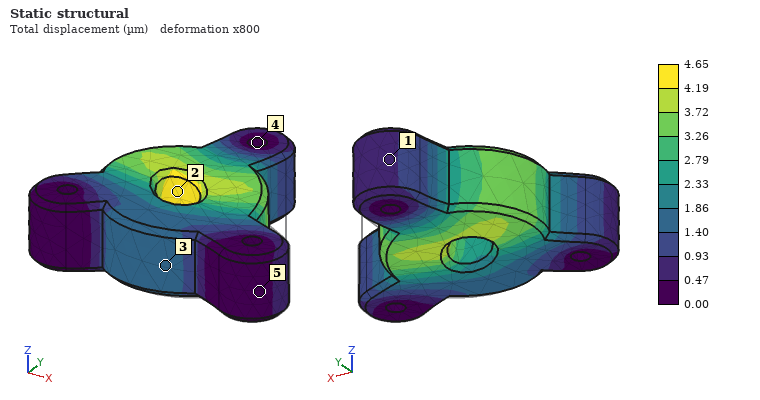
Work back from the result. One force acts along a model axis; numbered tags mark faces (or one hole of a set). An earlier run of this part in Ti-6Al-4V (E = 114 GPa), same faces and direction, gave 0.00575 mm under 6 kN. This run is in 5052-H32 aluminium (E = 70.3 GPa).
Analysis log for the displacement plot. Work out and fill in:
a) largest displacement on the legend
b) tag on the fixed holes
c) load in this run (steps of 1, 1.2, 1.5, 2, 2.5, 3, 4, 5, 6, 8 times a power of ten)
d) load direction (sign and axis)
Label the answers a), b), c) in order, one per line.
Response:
a) 4.65 µm
b) 4
c) 3 kN
d) -X
